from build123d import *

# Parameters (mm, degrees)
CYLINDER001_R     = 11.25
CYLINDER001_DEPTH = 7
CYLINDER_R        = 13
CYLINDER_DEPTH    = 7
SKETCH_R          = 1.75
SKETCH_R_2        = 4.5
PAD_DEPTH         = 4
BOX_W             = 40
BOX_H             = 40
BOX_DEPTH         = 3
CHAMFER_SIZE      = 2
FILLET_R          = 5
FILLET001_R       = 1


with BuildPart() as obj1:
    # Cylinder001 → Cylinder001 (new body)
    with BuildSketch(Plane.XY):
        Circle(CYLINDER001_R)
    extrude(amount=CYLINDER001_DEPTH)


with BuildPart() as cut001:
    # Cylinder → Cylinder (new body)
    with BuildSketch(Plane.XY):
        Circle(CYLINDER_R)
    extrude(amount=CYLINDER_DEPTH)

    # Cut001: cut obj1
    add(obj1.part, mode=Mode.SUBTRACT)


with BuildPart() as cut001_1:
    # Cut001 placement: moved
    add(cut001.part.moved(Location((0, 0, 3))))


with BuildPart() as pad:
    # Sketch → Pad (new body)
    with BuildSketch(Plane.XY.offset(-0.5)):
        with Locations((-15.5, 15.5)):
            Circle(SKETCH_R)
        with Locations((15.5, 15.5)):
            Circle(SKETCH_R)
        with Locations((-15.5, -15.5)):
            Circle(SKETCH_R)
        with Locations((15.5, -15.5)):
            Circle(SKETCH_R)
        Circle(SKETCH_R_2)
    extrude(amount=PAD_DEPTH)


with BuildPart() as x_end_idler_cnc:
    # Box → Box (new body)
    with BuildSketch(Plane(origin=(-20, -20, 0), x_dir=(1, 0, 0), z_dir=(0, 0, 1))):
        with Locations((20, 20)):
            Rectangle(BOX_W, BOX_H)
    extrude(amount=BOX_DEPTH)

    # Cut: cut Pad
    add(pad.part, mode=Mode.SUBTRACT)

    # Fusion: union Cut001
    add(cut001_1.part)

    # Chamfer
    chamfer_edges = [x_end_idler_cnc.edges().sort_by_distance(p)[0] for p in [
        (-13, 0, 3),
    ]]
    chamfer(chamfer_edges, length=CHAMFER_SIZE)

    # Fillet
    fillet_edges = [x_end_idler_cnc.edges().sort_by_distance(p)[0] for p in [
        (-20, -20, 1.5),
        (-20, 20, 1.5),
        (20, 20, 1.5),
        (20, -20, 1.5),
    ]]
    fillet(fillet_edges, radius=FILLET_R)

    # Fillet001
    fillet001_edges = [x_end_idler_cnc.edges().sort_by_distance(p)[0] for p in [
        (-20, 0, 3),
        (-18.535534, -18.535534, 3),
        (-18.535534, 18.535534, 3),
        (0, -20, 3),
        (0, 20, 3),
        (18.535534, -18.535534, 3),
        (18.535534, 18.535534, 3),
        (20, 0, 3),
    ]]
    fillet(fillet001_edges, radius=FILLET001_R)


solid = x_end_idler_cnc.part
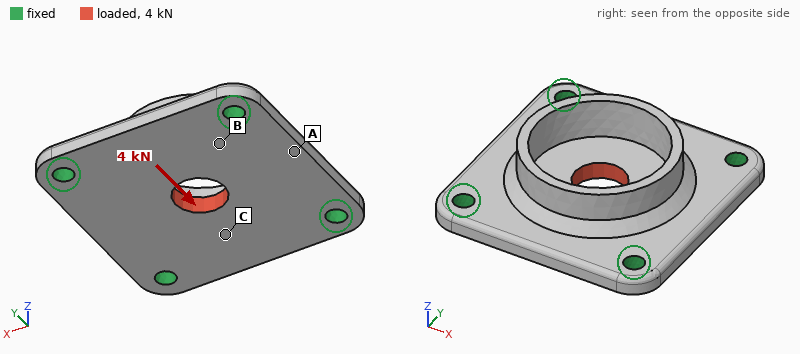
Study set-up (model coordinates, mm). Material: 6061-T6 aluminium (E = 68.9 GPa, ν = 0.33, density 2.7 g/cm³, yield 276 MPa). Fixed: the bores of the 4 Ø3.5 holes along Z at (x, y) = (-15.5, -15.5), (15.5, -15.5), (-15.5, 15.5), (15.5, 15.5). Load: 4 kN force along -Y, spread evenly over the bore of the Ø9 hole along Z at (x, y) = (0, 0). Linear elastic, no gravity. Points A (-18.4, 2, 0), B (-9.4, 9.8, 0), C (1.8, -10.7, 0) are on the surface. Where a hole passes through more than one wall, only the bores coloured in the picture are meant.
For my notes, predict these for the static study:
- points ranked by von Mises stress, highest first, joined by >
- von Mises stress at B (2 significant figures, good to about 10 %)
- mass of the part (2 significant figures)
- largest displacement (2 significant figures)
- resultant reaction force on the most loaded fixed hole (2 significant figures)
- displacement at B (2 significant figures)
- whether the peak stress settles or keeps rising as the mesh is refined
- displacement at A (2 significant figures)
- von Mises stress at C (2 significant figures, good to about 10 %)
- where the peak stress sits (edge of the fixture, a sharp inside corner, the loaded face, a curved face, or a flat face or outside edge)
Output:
B > C > A
38 MPa
15 g
13 µm
1.1 kN
5.5 µm
keeps rising
2.5 µm
19 MPa
edge of the fixture
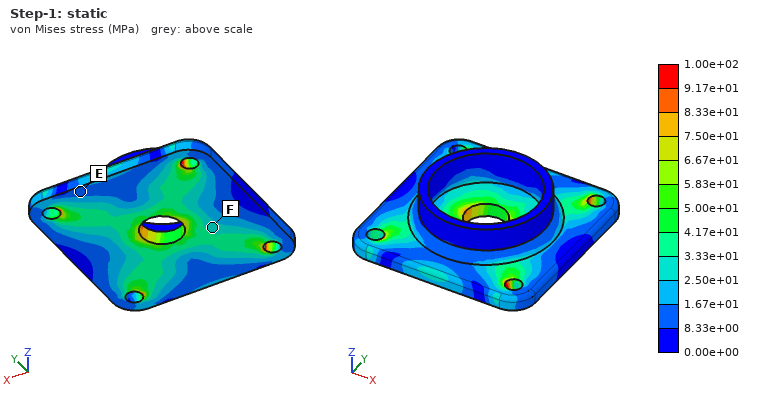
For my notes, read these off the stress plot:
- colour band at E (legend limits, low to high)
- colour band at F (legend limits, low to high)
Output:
8.33e+00 to 1.67e+01 MPa
2.50e+01 to 3.33e+01 MPa
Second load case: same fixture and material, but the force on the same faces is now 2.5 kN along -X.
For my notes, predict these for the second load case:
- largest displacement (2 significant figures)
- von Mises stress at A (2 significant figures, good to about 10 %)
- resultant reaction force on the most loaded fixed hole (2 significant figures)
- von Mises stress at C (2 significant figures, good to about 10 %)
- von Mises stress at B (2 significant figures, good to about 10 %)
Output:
8.2 µm
8.9 MPa
690 N
14 MPa
23 MPa
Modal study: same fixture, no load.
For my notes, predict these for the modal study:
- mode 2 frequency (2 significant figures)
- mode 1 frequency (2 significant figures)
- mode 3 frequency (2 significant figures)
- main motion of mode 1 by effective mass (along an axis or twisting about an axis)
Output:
19 kHz
14 kHz
19 kHz
along Z
